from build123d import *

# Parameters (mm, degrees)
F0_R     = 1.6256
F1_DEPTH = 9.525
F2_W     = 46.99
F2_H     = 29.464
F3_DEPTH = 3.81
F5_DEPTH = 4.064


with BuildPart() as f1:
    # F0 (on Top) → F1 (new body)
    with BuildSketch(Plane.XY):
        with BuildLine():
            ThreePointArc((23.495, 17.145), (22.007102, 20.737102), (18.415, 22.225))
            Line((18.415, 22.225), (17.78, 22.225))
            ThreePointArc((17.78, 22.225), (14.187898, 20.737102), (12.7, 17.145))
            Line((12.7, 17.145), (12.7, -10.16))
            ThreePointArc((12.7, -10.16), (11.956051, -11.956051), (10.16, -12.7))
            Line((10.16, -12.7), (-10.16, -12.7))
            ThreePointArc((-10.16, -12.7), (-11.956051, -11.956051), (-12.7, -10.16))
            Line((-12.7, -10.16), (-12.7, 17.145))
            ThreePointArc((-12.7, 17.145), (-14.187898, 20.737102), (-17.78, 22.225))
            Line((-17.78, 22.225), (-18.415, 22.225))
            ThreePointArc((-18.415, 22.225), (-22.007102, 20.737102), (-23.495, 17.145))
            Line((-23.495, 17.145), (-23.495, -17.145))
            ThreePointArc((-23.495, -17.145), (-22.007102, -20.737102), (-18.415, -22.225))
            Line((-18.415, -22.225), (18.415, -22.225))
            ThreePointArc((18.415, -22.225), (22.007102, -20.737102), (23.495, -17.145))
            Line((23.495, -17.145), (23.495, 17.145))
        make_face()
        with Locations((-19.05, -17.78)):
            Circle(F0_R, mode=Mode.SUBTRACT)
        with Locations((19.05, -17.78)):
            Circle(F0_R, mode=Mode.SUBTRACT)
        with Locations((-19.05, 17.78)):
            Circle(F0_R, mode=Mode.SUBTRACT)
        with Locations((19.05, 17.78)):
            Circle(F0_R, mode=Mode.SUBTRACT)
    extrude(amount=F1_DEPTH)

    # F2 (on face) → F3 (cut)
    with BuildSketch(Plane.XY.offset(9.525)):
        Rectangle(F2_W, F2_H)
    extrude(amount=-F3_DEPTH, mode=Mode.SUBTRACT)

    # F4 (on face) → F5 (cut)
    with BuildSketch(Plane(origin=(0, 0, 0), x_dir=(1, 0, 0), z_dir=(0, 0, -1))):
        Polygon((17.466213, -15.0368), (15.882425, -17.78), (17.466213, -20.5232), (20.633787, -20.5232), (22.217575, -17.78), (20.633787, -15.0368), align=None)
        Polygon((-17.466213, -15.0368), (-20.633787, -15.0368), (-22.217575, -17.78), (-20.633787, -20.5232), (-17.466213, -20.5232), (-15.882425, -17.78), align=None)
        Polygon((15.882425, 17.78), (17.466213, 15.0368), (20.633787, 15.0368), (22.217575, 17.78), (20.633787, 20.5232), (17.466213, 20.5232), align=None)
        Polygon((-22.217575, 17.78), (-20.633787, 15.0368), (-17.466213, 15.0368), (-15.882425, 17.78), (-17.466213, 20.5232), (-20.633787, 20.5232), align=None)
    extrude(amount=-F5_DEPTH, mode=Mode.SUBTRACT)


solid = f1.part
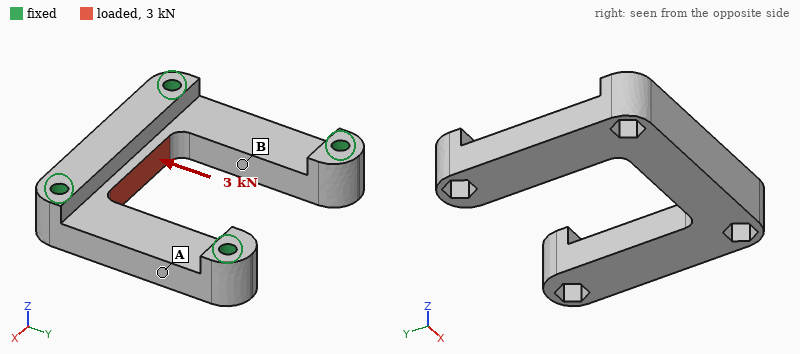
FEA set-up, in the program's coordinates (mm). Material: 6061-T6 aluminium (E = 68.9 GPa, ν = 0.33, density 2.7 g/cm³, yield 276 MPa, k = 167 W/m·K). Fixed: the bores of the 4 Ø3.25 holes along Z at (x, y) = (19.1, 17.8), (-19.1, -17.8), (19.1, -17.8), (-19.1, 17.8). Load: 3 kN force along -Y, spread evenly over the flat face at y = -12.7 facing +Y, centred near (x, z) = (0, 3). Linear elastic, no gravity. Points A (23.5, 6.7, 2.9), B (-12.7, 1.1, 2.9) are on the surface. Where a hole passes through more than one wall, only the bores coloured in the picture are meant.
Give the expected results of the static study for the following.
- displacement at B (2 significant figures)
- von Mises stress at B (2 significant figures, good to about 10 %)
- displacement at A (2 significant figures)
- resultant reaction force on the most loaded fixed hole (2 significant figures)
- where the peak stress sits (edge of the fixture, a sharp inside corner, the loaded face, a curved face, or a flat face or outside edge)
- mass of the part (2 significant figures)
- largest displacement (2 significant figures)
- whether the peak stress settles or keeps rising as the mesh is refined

9.1 µm
29 MPa
8.0 µm
980 N
edge of the fixture
21 g
40 µm
keeps rising
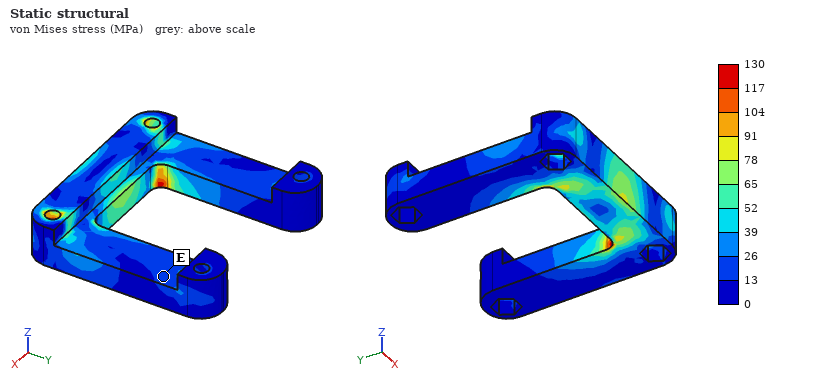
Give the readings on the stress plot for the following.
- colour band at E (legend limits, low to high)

13 to 26 MPa
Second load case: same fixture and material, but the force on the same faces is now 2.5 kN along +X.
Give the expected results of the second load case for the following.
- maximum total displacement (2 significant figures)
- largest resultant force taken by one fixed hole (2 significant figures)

7.9 µm
1.3 kN
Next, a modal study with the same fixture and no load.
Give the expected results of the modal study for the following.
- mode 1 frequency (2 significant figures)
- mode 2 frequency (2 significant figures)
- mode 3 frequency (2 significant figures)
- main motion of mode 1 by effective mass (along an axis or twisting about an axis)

18 kHz
19 kHz
20 kHz
along Z
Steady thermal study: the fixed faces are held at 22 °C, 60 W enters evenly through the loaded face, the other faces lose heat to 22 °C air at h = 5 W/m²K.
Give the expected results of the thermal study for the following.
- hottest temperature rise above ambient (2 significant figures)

42 K
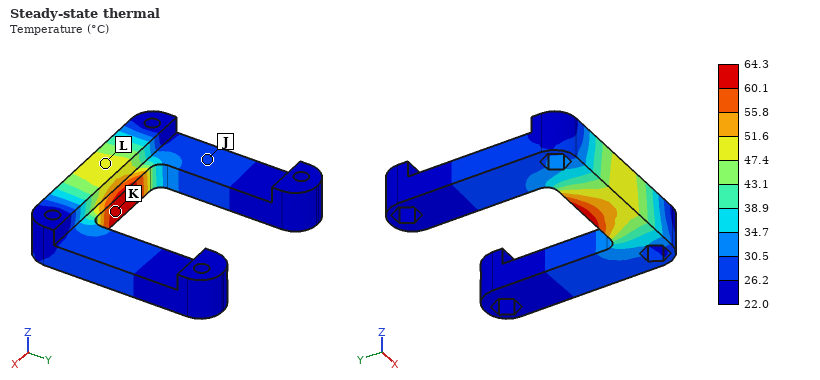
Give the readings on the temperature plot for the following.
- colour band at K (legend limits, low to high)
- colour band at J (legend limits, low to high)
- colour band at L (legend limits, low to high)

60.1 to 64.3 °C
26.2 to 30.5 °C
47.4 to 51.6 °C
